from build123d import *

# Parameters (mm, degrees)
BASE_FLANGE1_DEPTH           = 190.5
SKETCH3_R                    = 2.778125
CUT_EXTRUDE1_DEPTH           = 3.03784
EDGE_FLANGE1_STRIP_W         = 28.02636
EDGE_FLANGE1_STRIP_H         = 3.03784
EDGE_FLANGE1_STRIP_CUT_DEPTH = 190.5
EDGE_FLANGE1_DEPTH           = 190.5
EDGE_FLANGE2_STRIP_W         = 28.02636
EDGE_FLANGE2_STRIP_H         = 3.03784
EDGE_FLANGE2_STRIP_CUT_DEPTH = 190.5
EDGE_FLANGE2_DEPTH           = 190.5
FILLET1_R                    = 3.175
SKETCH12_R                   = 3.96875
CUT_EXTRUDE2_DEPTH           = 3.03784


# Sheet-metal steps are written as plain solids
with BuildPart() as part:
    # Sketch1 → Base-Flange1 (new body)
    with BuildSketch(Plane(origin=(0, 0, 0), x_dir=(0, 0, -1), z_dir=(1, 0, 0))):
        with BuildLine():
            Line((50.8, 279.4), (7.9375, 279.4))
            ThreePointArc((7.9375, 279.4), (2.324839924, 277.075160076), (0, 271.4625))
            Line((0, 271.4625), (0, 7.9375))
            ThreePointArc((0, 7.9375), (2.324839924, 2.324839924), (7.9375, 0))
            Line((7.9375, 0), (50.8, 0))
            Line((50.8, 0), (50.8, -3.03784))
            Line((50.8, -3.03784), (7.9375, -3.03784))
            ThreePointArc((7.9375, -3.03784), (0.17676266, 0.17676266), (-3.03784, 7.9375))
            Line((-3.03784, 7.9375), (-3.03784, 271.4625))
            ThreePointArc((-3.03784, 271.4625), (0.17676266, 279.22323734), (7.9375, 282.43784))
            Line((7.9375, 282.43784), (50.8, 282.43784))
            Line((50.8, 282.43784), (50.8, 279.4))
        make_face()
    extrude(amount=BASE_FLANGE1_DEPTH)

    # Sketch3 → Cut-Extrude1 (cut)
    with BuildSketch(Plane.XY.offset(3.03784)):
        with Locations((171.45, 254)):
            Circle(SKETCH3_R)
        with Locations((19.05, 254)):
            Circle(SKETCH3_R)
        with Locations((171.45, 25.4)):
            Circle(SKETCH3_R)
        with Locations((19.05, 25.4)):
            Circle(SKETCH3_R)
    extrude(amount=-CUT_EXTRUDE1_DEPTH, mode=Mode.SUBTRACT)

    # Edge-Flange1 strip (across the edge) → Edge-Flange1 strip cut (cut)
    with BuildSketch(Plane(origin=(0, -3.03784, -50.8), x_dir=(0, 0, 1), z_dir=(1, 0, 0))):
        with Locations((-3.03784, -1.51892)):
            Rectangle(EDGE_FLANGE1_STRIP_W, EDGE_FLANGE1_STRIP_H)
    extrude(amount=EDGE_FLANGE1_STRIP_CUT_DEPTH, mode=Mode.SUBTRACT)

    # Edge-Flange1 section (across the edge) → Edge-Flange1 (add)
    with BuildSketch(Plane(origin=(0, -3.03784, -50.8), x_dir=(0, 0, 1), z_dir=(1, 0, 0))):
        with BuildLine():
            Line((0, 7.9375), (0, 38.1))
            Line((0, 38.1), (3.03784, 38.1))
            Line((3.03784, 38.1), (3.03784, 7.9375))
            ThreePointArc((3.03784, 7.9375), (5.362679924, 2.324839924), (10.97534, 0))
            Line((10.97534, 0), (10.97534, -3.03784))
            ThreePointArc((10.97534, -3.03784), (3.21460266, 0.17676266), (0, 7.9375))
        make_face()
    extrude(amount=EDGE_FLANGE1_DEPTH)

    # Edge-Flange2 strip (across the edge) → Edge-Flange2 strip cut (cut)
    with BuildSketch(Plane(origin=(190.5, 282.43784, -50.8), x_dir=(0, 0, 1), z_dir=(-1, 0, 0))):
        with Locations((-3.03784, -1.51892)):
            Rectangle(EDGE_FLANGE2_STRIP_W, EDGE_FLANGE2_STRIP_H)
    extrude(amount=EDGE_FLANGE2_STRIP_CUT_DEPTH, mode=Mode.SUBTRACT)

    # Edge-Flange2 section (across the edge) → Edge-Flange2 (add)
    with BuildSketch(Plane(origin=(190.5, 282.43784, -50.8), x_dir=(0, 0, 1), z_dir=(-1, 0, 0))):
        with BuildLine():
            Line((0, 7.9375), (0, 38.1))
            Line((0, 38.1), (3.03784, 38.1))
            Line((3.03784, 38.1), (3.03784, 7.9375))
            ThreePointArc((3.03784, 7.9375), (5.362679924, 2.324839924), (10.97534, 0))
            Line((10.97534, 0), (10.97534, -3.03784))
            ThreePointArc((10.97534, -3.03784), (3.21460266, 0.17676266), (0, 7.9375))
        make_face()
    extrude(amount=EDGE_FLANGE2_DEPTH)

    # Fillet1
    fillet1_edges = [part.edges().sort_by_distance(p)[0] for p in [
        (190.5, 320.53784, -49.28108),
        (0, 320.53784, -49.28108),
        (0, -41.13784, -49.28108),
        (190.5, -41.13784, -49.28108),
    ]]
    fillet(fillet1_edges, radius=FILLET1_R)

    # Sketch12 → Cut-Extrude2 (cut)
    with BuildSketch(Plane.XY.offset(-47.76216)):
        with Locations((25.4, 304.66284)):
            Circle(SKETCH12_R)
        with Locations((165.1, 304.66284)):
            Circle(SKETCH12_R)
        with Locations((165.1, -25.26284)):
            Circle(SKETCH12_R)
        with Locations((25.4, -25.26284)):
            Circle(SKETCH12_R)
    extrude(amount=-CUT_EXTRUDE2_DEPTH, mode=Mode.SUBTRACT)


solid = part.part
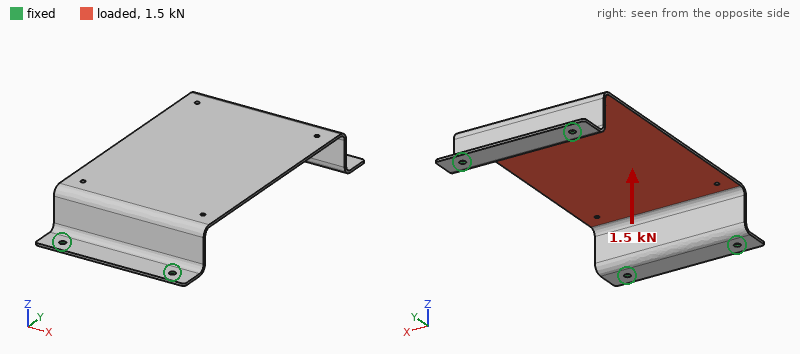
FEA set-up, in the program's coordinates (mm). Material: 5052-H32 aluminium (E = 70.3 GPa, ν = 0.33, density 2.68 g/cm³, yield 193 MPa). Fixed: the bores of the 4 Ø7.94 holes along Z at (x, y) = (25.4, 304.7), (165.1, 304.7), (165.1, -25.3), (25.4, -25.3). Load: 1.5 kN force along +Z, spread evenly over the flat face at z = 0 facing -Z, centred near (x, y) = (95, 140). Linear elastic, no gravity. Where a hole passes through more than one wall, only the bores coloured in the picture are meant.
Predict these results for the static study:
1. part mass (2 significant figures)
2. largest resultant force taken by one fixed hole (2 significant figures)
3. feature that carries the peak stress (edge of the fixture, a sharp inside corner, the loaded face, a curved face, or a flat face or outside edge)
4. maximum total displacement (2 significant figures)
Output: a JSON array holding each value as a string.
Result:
["690 g", "640 N", "a curved face", "3.8 mm"]
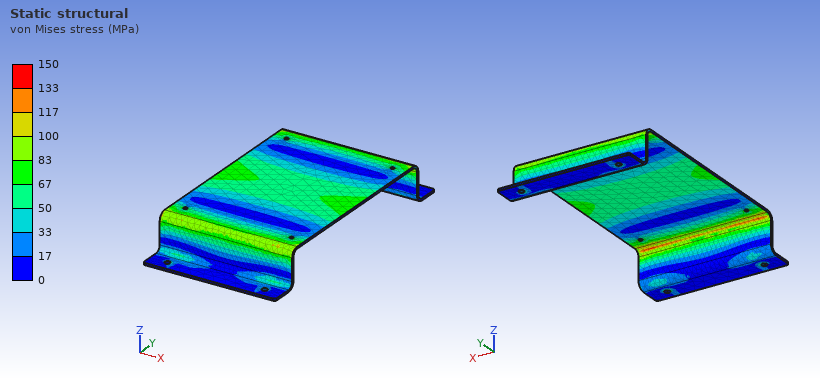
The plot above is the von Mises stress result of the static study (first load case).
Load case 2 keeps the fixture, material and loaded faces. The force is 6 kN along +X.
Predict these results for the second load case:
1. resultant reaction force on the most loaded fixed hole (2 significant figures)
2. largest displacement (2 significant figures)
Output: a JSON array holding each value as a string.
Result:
["1.9 kN", "0.38 mm"]
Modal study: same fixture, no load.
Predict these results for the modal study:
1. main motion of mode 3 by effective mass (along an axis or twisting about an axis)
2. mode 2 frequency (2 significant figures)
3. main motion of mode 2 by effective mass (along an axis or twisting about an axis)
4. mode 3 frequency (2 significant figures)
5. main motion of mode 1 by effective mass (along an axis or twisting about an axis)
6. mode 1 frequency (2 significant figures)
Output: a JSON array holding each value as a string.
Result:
["twisting about Y", "230 Hz", "along Y", "270 Hz", "along Z", "190 Hz"]
